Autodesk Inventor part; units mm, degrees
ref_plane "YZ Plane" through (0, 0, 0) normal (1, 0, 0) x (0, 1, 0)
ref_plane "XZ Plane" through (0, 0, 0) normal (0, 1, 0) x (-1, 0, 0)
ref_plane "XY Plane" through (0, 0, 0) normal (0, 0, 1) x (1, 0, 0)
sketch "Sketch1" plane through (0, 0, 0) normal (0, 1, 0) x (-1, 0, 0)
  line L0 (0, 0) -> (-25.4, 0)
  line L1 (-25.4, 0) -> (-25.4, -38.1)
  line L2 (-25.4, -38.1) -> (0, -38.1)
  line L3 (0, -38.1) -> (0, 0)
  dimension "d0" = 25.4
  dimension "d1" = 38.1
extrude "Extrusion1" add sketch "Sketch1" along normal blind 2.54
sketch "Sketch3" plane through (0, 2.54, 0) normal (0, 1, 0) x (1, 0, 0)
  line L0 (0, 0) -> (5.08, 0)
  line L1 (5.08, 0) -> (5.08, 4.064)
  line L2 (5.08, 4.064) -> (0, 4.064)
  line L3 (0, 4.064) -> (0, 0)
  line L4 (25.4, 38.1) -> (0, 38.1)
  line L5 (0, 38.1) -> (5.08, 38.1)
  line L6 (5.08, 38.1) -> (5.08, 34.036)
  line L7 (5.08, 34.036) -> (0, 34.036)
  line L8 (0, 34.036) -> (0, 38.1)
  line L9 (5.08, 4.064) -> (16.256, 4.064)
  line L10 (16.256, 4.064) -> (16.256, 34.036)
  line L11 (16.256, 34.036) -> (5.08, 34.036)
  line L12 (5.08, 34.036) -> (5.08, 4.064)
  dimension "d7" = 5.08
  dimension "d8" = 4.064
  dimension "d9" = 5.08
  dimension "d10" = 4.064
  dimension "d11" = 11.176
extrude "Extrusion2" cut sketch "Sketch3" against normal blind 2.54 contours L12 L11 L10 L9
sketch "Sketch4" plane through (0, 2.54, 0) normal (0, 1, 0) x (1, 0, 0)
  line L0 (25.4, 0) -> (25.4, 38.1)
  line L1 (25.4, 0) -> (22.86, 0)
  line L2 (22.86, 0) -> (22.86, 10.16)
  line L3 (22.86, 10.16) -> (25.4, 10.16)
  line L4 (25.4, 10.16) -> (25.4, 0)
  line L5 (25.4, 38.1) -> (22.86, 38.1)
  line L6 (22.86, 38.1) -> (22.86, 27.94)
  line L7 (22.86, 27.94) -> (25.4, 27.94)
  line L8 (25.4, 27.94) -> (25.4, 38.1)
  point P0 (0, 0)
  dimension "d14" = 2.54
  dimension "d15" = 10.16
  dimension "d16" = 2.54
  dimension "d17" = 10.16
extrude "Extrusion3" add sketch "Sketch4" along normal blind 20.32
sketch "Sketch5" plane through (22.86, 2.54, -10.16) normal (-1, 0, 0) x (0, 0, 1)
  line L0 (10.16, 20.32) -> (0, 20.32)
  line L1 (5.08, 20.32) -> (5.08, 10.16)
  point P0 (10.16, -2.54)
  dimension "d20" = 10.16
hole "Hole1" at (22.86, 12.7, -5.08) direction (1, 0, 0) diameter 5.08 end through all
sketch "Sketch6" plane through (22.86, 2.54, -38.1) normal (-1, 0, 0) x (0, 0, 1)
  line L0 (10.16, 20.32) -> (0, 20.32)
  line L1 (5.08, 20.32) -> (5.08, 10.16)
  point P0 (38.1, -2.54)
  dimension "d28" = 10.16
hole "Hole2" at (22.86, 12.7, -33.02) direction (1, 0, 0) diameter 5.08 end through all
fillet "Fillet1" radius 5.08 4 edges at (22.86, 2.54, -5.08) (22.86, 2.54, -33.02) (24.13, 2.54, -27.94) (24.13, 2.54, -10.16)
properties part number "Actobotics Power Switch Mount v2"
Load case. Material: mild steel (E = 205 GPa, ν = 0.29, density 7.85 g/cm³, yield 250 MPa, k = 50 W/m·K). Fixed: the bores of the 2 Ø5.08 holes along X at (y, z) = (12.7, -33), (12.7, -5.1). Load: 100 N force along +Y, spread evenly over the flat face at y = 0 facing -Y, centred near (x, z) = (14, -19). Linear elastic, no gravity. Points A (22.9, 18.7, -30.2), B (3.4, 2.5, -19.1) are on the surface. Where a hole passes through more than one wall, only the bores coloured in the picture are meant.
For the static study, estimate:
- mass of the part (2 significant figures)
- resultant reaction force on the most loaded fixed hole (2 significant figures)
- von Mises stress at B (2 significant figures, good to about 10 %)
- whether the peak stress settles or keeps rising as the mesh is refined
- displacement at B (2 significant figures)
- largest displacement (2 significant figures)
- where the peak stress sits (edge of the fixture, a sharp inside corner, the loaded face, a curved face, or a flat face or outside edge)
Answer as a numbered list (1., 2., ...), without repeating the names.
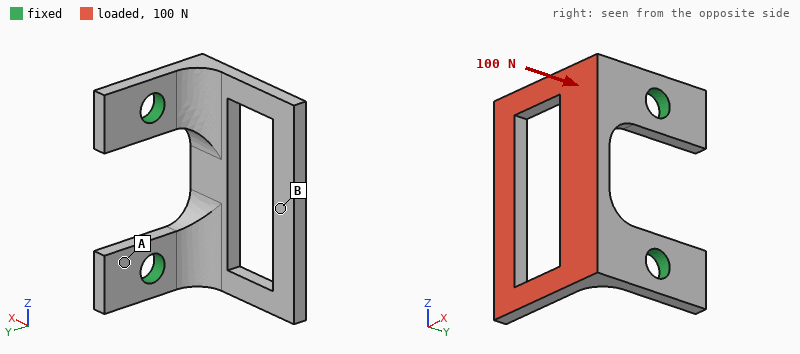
1. 21 g
2. 50 N
3. 14 MPa
4. keeps rising
5. 53 µm
6. 65 µm
7. a sharp inside corner
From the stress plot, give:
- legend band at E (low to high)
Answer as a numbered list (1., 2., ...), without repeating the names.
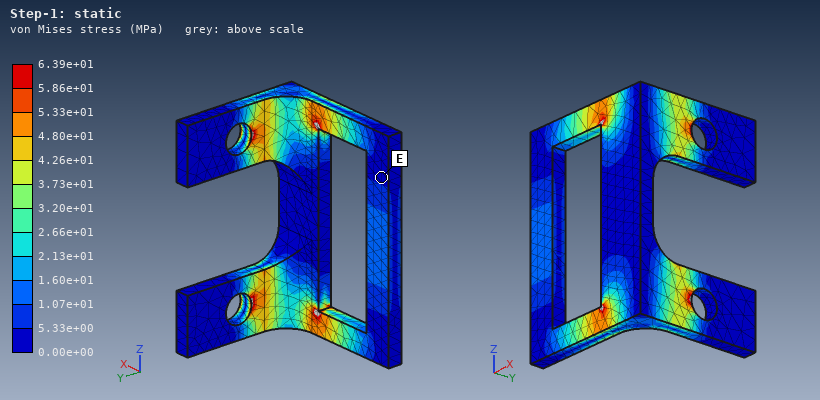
1. 0.00e+00 to 5.33e+00 MPa
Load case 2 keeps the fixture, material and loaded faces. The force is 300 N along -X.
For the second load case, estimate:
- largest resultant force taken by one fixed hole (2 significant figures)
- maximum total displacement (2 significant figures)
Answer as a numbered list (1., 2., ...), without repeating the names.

1. 150 N
2. 77 µm
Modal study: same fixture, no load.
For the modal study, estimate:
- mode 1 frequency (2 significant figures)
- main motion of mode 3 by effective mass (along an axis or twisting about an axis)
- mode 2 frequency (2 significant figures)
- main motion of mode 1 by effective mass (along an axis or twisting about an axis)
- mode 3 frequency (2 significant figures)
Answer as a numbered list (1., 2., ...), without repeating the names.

1. 2100 Hz
2. along Z
3. 4400 Hz
4. along Y
5. 6400 Hz
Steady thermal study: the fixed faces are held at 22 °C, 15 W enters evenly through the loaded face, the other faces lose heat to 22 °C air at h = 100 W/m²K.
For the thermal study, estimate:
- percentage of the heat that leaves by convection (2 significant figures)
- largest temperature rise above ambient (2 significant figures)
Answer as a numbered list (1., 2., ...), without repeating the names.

1. 41 %
2. 76 K
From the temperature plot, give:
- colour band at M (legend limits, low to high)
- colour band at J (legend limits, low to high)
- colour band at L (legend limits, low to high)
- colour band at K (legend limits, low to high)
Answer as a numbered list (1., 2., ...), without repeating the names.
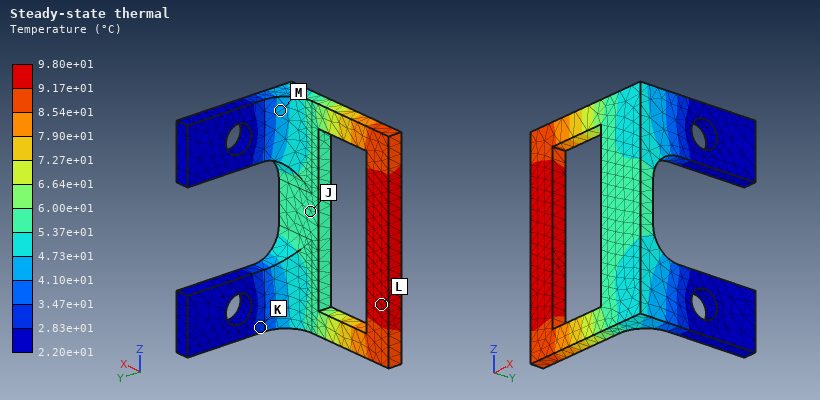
1. 4.10e+01 to 4.73e+01 °C
2. 5.37e+01 to 6.00e+01 °C
3. 9.17e+01 to 9.80e+01 °C
4. 2.83e+01 to 3.47e+01 °C
